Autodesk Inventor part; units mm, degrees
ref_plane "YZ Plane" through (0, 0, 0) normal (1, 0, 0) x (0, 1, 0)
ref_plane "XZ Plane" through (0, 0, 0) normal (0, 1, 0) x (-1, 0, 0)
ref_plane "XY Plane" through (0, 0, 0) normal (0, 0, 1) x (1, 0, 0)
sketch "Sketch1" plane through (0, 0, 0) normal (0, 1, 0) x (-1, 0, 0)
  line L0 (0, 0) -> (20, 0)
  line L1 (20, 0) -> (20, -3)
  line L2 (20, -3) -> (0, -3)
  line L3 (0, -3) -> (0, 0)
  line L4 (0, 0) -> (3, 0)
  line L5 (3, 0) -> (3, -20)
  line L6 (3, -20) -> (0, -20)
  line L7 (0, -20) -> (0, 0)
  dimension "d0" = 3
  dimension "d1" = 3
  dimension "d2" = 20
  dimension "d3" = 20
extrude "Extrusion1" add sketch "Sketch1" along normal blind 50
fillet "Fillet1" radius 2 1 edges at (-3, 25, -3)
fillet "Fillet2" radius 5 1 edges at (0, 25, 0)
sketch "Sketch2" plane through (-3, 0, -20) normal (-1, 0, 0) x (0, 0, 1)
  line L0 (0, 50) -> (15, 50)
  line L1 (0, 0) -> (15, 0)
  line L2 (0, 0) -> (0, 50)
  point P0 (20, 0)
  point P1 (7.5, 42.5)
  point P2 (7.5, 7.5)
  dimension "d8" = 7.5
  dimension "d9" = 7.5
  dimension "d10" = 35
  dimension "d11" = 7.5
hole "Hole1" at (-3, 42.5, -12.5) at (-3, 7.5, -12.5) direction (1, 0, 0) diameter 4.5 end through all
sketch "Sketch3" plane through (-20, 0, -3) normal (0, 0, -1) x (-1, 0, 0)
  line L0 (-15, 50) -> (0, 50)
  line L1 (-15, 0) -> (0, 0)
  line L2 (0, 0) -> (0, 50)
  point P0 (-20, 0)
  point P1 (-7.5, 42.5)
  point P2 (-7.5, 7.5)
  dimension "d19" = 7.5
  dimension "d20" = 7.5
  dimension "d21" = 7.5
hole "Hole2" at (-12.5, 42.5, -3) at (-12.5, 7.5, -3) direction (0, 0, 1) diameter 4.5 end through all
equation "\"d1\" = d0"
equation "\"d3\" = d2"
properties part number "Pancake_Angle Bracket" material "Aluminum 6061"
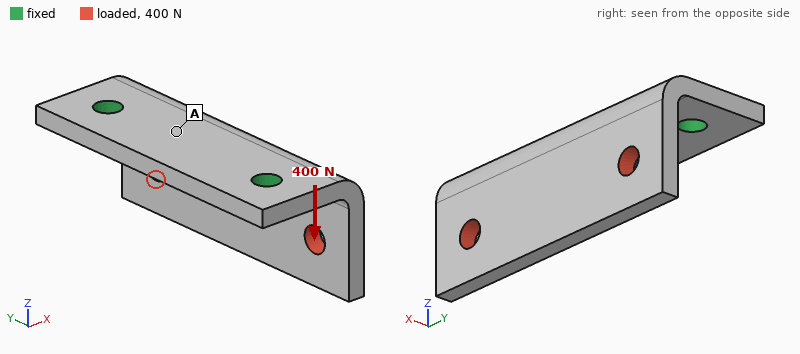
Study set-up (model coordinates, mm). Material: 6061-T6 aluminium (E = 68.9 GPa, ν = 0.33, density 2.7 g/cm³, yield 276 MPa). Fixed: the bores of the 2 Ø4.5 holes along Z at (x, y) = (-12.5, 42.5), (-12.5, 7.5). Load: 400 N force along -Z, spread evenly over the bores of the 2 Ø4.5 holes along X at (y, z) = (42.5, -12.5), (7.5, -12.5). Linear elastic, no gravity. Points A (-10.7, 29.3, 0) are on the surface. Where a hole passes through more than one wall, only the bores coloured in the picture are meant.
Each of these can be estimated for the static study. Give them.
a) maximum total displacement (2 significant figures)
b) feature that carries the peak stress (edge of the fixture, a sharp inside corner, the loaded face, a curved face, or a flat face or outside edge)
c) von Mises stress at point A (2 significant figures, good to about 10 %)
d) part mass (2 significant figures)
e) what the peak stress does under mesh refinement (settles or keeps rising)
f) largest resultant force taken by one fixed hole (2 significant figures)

69 µm
edge of the fixture
13 MPa
14 g
keeps rising
200 N
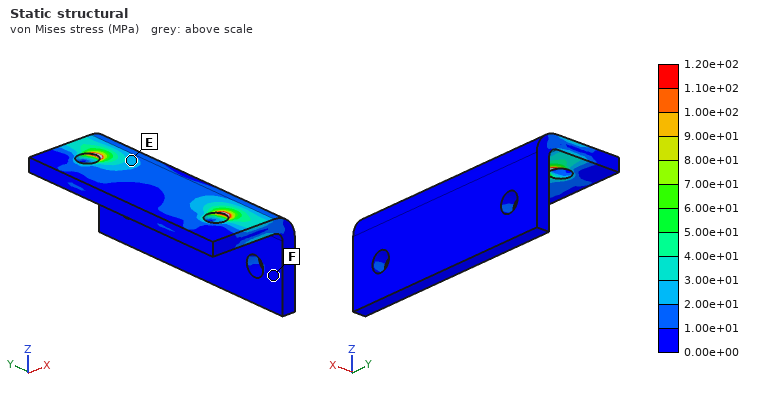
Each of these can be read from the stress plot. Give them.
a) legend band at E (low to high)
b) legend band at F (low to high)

2.00e+01 to 3.00e+01 MPa
0.00e+00 to 1.00e+01 MPa
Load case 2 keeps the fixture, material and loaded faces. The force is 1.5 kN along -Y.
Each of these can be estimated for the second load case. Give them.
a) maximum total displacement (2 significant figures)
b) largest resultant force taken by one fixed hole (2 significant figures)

0.10 mm
960 N
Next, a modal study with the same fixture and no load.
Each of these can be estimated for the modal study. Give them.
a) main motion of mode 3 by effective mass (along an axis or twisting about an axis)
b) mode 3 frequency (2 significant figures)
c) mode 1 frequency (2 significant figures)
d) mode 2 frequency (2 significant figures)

along Z
11 kHz
3800 Hz
6200 Hz
